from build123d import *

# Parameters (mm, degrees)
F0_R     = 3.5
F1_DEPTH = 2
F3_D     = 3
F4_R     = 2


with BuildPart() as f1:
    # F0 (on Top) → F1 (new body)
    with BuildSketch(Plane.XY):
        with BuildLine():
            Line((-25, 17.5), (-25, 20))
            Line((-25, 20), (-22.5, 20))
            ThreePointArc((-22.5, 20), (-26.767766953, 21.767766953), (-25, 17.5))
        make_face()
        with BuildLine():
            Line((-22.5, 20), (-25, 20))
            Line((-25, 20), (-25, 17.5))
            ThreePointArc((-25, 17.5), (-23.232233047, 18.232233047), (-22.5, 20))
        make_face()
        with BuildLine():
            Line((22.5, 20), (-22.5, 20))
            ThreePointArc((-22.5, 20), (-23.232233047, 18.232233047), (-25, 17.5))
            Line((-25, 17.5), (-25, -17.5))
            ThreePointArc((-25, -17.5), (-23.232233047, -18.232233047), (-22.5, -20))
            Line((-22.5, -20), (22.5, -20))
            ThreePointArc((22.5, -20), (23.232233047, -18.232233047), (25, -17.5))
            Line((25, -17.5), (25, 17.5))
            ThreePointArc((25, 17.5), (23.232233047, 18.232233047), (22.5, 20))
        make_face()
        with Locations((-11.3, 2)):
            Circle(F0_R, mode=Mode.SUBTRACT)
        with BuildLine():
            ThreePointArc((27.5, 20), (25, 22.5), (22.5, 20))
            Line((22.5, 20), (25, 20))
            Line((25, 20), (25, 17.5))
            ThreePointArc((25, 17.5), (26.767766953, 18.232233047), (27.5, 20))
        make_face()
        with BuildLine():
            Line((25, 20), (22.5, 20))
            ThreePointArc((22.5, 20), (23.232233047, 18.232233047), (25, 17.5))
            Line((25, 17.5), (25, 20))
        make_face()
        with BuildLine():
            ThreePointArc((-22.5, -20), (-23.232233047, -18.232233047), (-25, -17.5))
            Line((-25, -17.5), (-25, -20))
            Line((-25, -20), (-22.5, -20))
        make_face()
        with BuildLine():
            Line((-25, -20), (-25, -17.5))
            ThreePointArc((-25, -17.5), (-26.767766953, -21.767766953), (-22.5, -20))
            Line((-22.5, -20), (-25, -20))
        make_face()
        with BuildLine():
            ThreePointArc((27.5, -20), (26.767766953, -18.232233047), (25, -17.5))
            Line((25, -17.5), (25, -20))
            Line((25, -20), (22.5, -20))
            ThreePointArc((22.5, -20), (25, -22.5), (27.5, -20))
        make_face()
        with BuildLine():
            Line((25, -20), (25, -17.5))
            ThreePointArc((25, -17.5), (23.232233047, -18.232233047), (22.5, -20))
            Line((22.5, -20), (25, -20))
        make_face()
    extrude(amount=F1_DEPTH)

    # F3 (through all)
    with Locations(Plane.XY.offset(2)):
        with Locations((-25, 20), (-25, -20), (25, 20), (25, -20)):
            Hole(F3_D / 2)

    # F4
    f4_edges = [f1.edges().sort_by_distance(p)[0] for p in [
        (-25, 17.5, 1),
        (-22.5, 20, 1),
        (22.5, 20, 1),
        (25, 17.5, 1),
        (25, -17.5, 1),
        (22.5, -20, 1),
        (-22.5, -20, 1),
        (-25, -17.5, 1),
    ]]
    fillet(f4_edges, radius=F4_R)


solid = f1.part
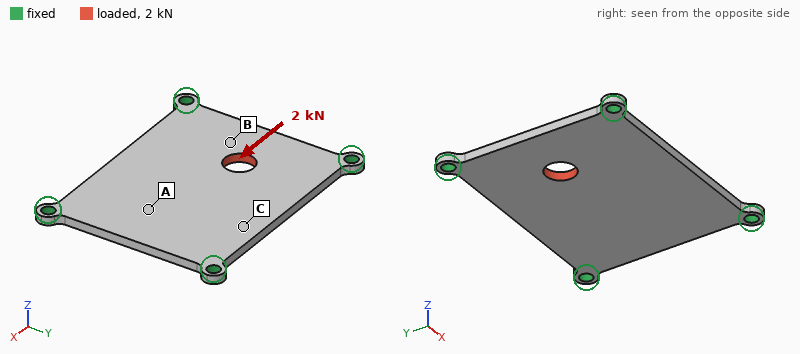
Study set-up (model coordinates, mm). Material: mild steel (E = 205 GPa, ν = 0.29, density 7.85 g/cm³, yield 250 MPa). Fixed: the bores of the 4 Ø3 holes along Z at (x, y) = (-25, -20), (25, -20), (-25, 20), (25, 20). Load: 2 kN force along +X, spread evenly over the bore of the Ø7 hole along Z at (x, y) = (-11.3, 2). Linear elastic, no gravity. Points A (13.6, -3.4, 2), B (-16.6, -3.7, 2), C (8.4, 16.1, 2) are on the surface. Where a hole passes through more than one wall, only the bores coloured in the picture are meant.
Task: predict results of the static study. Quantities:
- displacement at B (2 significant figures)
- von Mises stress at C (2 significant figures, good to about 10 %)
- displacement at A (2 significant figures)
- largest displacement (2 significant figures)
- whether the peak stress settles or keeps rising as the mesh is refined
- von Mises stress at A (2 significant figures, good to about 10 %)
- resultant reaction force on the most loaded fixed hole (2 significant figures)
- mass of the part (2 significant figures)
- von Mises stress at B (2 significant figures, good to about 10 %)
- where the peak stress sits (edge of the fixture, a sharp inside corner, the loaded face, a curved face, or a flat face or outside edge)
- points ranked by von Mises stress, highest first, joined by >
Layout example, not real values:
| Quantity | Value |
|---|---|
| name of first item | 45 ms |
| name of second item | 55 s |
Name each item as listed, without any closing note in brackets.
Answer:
| Quantity | Value |
|---|---|
| displacement at B | 5.1 µm |
| von Mises stress at C | 18 MPa |
| displacement at A | 2.9 µm |
| largest displacement | 6.8 µm |
| whether the peak stress settles or keeps rising as the mesh is refined | keeps rising |
| von Mises stress at A | 8.2 MPa |
| resultant reaction force on the most loaded fixed hole | 680 N |
| mass of the part | 31 g |
| von Mises stress at B | 33 MPa |
| where the peak stress sits | edge of the fixture |
| points ranked by von Mises stress, highest first, joined by > | B > C > A |
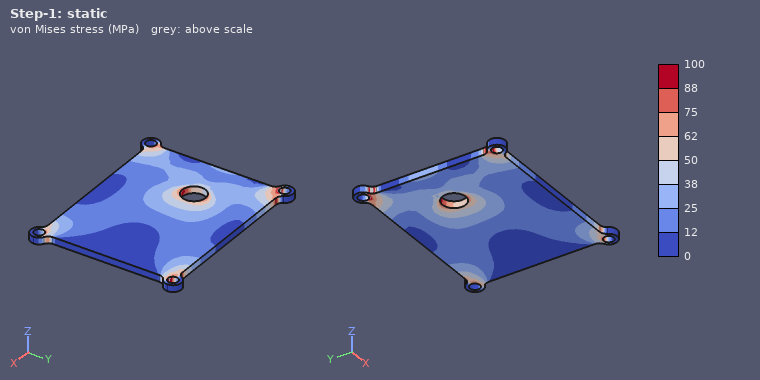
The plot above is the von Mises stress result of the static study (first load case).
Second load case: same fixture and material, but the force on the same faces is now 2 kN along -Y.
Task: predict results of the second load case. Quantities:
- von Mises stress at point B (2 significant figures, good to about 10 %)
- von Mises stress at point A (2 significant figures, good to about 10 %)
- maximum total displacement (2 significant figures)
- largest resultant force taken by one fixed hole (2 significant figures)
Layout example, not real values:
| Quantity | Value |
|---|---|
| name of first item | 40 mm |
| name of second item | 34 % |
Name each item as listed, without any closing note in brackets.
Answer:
| Quantity | Value |
|---|---|
| von Mises stress at point B | 39 MPa |
| von Mises stress at point A | 13 MPa |
| maximum total displacement | 6.6 µm |
| largest resultant force taken by one fixed hole | 790 N |
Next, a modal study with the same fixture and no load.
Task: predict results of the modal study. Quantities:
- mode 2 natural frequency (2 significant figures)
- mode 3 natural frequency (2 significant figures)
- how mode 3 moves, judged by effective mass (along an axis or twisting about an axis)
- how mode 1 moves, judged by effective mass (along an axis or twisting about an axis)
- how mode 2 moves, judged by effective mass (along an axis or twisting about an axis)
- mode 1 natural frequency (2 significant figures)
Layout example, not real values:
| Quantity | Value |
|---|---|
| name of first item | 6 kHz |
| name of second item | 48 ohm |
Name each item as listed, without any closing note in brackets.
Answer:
| Quantity | Value |
|---|---|
| mode 2 natural frequency | 5200 Hz |
| mode 3 natural frequency | 6300 Hz |
| how mode 3 moves, judged by effective mass | twisting about Y |
| how mode 1 moves, judged by effective mass | along Z |
| how mode 2 moves, judged by effective mass | twisting about X |
| mode 1 natural frequency | 2900 Hz |
